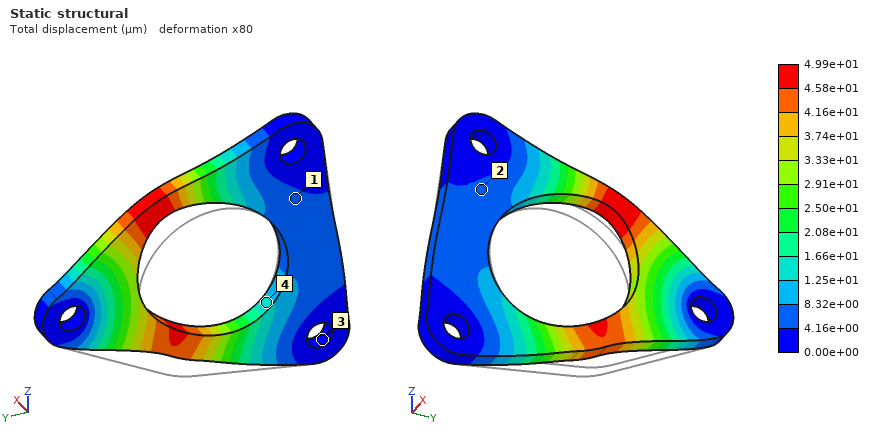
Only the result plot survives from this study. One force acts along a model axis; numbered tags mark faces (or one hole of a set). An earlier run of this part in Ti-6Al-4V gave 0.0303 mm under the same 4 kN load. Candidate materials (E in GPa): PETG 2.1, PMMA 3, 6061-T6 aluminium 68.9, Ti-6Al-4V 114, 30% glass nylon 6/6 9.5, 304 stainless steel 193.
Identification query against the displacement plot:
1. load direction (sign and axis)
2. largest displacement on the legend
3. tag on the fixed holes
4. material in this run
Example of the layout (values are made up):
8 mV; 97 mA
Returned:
+Z; 4.99e+01 µm; 3; 6061-T6 aluminium
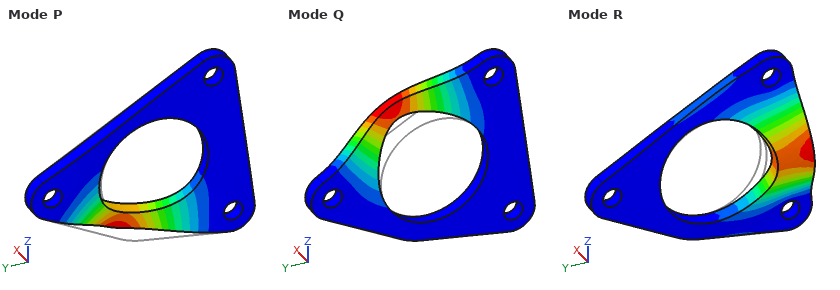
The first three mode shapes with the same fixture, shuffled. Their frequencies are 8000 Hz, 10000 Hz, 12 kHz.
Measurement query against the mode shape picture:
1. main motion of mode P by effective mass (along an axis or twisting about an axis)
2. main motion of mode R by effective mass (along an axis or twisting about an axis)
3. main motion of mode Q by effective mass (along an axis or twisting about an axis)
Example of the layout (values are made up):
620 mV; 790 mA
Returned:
along X; along X; along X
